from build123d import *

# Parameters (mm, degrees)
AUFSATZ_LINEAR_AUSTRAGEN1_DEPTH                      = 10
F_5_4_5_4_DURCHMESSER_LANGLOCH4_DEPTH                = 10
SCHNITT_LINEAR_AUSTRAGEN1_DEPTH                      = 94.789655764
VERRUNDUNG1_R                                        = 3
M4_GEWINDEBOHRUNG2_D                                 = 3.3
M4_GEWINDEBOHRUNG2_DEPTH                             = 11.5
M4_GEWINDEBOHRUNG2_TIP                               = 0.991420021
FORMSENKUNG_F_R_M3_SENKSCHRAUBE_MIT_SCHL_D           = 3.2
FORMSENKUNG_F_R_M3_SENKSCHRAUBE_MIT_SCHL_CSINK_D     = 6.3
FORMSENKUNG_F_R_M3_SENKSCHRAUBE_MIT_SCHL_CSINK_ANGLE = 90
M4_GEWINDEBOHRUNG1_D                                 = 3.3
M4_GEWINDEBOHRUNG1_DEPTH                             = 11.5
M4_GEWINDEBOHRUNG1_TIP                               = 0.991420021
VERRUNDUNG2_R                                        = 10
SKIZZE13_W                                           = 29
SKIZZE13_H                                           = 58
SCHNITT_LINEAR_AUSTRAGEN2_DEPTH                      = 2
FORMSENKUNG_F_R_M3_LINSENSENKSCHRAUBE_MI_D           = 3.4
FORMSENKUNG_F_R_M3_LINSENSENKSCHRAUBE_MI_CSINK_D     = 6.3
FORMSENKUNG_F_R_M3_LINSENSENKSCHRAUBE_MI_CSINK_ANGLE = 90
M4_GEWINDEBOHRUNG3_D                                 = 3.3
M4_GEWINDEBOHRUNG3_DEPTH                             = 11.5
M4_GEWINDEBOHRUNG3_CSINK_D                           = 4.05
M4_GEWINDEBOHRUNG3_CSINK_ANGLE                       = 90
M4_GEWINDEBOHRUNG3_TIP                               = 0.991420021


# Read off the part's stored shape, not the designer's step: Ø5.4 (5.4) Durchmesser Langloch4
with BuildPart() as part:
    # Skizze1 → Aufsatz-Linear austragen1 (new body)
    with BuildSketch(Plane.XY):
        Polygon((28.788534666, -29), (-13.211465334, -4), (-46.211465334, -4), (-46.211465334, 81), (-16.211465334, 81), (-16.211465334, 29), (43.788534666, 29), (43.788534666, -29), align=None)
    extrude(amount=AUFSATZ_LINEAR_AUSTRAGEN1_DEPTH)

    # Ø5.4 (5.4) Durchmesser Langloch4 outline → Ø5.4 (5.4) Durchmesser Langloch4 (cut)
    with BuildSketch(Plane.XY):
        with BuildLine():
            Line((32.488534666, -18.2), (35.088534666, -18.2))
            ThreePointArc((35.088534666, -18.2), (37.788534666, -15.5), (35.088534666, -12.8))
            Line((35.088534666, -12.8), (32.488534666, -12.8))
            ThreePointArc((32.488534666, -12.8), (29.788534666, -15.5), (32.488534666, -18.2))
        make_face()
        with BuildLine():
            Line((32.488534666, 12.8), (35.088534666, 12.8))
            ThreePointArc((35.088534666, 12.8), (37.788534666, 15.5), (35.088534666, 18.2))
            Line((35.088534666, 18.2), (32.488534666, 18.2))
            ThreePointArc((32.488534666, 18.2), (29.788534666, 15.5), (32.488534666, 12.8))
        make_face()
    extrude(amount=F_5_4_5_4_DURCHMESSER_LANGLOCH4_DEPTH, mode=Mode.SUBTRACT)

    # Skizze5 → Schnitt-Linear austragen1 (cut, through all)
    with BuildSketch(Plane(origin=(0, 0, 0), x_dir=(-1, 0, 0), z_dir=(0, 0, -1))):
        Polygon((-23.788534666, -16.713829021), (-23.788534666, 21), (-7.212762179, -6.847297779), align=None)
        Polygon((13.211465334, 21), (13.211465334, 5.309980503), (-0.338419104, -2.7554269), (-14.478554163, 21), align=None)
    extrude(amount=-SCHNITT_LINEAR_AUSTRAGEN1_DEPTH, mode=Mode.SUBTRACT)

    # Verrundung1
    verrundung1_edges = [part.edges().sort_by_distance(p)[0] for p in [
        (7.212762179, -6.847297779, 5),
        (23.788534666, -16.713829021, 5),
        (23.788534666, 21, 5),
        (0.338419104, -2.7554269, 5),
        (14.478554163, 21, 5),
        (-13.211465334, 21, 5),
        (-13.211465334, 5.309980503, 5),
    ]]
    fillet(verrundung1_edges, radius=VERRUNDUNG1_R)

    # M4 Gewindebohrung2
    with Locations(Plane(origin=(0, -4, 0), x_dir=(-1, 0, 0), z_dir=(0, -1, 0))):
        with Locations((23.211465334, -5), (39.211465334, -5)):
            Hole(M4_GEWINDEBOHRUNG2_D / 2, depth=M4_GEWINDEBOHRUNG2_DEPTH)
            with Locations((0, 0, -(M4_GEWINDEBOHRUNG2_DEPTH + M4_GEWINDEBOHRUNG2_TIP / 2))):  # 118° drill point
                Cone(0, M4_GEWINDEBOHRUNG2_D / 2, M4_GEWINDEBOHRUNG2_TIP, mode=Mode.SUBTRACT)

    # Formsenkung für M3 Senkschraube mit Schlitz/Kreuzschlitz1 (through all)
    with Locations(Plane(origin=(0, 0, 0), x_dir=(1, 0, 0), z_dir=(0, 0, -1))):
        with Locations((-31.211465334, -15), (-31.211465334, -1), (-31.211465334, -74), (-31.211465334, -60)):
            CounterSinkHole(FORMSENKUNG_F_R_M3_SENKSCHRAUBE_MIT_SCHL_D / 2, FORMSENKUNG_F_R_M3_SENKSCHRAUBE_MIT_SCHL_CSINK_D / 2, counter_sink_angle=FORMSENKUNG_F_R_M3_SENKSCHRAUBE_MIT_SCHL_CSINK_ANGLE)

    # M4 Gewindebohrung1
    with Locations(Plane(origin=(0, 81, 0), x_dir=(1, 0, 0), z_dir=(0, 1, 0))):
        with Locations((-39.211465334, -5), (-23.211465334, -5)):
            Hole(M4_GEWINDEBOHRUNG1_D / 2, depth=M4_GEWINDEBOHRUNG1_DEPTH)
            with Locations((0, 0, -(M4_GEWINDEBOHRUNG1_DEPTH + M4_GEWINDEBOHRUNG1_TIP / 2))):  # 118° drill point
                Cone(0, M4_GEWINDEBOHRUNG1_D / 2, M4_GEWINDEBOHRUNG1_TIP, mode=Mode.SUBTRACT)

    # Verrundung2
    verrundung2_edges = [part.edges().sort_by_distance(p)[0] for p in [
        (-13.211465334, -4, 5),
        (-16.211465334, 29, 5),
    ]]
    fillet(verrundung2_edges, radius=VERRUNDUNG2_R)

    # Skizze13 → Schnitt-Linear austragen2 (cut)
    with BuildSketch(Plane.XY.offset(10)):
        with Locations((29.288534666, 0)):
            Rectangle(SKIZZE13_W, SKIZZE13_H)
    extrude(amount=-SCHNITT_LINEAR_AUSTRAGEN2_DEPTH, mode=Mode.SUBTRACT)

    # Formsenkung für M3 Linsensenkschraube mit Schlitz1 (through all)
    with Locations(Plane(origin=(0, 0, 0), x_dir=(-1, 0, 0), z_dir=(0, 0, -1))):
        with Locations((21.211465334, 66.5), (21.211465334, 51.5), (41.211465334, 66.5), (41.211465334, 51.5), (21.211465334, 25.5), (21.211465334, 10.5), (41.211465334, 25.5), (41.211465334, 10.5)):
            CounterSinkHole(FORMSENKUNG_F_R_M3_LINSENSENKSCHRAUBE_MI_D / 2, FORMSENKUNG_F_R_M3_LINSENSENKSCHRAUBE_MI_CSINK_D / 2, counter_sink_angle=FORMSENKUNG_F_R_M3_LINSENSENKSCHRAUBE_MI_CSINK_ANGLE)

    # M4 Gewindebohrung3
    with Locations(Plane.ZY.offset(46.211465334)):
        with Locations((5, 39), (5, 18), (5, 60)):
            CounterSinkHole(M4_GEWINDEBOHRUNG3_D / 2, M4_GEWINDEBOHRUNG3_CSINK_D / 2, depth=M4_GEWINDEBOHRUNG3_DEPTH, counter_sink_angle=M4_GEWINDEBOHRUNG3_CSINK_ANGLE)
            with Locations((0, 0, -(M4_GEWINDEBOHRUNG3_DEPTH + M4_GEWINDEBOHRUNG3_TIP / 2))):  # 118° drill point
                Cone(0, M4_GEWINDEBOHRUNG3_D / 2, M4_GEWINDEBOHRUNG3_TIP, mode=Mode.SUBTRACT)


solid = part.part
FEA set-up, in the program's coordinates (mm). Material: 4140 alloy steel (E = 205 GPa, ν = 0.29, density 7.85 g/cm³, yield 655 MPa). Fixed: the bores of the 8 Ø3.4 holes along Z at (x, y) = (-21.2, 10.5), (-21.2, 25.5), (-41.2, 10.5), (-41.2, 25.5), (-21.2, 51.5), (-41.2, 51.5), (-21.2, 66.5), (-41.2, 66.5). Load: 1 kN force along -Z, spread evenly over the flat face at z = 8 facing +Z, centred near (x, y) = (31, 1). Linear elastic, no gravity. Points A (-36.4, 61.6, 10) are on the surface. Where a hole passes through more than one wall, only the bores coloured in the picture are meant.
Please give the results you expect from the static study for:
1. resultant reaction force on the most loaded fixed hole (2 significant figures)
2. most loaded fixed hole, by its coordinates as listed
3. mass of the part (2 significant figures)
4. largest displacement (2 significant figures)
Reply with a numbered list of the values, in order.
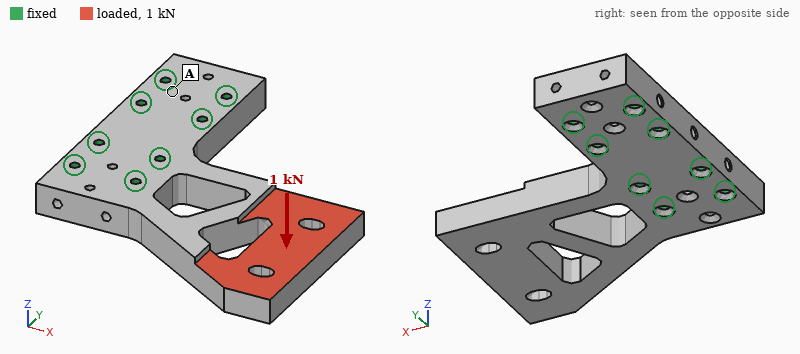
1. 1.6 kN
2. (-21.2, 10.5)
3. 330 g
4. 0.29 mm
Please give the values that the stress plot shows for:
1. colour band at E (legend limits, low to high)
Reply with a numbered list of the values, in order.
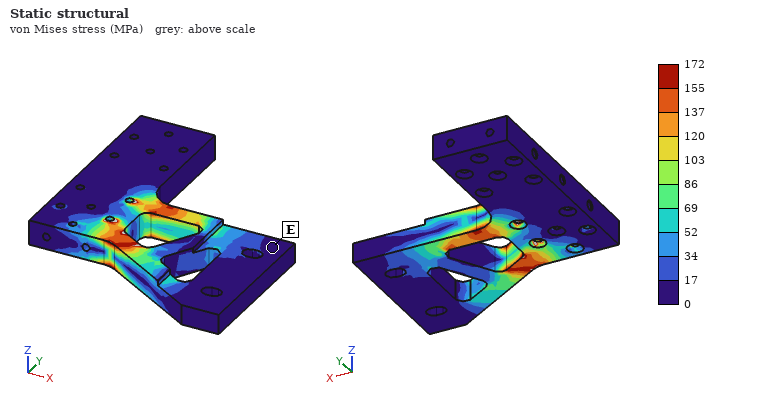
1. 0 to 17 MPa
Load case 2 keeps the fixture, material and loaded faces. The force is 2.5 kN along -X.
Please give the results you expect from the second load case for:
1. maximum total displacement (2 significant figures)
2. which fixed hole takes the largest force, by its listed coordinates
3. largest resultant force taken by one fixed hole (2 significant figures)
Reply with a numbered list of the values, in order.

1. 70 µm
2. (-21.2, 10.5)
3. 1.6 kN
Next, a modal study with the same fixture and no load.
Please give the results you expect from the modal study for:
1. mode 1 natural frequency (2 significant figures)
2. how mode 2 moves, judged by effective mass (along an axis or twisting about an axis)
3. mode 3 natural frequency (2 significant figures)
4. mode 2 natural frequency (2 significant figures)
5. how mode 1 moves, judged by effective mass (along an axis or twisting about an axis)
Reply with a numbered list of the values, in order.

1. 1200 Hz
2. along Y
3. 2800 Hz
4. 2700 Hz
5. along Z
